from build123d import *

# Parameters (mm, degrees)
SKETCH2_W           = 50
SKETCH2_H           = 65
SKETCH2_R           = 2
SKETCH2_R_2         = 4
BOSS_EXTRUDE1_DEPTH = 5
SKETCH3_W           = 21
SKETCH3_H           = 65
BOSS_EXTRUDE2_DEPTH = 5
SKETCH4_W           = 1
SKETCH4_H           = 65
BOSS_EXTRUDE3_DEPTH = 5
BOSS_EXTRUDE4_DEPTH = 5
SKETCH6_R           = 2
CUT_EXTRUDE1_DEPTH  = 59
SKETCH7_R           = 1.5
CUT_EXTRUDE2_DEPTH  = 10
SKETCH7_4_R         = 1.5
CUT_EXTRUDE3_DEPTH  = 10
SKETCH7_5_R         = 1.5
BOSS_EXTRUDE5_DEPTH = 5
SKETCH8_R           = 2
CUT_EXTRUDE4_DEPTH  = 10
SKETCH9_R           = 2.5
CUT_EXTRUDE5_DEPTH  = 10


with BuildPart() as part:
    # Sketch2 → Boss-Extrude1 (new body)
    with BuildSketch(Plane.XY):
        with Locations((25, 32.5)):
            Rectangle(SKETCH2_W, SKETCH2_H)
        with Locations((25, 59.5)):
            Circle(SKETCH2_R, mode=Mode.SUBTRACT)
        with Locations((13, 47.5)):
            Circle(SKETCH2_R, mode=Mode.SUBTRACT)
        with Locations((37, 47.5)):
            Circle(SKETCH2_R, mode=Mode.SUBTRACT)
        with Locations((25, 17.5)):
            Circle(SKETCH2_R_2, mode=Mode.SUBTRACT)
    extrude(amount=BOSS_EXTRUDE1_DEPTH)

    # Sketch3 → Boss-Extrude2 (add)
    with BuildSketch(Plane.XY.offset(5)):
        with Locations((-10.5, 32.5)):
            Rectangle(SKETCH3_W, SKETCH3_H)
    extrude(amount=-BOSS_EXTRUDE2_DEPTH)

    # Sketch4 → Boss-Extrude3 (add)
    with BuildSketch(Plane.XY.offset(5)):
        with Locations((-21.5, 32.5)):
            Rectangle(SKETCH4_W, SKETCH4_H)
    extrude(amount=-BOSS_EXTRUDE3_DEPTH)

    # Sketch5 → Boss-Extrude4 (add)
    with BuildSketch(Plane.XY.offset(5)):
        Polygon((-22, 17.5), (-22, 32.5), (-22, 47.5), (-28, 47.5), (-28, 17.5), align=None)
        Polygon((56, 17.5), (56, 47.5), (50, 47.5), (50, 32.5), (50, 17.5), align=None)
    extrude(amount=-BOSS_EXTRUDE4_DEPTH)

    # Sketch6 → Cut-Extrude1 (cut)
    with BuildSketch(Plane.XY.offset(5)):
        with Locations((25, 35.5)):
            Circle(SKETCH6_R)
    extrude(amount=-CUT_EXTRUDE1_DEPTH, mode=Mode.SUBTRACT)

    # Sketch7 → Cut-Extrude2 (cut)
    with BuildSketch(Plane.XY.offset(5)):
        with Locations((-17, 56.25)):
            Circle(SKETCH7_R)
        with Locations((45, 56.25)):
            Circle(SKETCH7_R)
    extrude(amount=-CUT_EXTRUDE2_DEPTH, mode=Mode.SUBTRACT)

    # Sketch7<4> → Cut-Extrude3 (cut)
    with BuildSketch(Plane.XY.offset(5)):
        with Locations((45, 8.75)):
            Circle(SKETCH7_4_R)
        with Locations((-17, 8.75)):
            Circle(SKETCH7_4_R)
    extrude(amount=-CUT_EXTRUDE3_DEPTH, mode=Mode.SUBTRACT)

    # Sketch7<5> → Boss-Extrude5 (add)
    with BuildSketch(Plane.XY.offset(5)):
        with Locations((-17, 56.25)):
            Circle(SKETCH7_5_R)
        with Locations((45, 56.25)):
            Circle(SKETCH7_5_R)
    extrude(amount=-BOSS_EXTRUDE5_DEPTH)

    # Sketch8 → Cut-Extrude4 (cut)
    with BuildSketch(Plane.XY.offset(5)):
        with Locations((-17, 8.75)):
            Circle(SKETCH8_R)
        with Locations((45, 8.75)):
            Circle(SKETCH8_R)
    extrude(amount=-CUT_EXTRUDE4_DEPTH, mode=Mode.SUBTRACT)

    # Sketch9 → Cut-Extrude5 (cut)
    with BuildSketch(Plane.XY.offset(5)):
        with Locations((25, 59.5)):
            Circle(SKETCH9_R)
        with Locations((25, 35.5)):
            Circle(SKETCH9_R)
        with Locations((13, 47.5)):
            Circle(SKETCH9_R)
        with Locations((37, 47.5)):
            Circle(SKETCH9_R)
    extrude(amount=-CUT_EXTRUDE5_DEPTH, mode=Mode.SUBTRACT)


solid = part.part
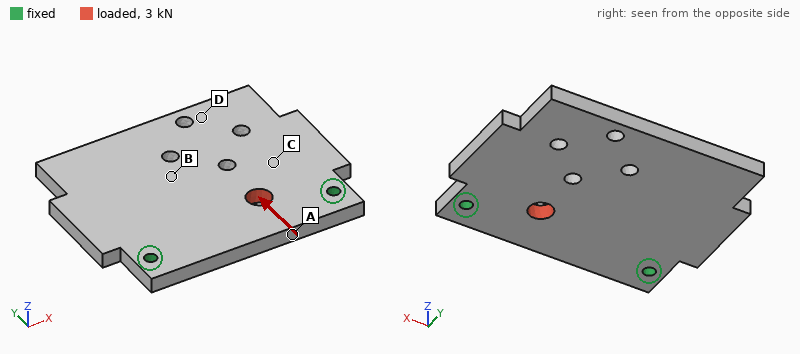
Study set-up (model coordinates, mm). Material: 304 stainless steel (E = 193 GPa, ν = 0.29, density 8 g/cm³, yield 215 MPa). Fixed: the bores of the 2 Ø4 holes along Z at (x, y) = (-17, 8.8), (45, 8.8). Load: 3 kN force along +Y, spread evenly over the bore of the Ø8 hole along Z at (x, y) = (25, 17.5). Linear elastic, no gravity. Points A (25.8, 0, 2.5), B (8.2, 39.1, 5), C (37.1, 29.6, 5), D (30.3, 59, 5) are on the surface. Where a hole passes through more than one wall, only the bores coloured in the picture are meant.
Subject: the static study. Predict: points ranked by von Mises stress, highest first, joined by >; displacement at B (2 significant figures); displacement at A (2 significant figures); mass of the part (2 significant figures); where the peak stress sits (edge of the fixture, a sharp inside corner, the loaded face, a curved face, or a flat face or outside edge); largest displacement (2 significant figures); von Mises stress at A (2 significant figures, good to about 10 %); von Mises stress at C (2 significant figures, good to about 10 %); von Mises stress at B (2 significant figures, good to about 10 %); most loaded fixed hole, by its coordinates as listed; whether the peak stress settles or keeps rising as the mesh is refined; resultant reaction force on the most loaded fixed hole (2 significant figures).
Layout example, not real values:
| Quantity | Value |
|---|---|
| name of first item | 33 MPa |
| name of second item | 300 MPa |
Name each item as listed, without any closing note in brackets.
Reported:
| Quantity | Value |
|---|---|
| points ranked by von Mises stress, highest first, joined by > | A > C > B > D |
| displacement at B | 2.7 µm |
| displacement at A | 4.1 µm |
| mass of the part | 200 g |
| where the peak stress sits | edge of the fixture |
| largest displacement | 5.1 µm |
| von Mises stress at A | 25 MPa |
| von Mises stress at C | 13 MPa |
| von Mises stress at B | 7.7 MPa |
| most loaded fixed hole, by its coordinates as listed | (45, 8.8) |
| whether the peak stress settles or keeps rising as the mesh is refined | keeps rising |
| resultant reaction force on the most loaded fixed hole | 2.1 kN |
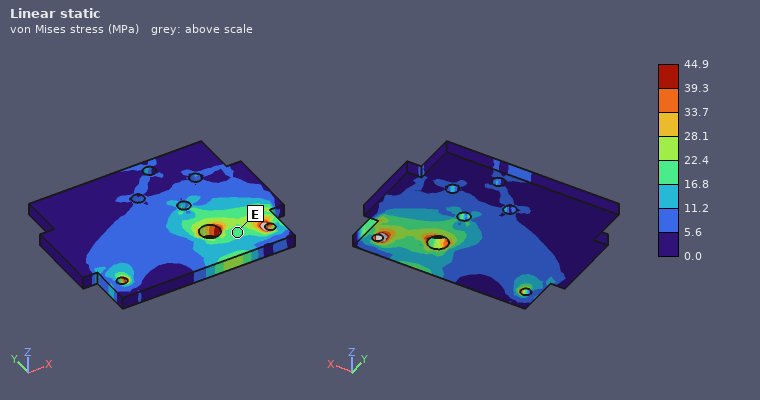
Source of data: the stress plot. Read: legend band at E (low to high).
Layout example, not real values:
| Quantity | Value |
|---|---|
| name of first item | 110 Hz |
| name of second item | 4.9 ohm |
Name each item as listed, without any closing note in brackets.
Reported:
| Quantity | Value |
|---|---|
| legend band at E | 16.8 to 22.4 MPa |
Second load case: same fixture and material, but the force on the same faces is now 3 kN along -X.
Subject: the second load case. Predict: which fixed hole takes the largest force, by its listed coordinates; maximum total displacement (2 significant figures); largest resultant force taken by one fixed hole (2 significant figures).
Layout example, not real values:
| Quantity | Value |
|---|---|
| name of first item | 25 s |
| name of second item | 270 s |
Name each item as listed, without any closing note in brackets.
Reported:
| Quantity | Value |
|---|---|
| which fixed hole takes the largest force, by its listed coordinates | (45, 8.8) |
| maximum total displacement | 3.4 µm |
| largest resultant force taken by one fixed hole | 1.8 kN |
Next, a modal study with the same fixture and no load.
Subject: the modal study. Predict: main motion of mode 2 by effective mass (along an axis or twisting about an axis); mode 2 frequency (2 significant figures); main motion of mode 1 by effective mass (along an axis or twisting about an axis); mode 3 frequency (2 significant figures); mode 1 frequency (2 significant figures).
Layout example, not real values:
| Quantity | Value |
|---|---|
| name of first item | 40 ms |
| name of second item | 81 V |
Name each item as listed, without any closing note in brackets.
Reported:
| Quantity | Value |
|---|---|
| main motion of mode 2 by effective mass | twisting about Y |
| mode 2 frequency | 2400 Hz |
| main motion of mode 1 by effective mass | along Z |
| mode 3 frequency | 5000 Hz |
| mode 1 frequency | 1000 Hz |
